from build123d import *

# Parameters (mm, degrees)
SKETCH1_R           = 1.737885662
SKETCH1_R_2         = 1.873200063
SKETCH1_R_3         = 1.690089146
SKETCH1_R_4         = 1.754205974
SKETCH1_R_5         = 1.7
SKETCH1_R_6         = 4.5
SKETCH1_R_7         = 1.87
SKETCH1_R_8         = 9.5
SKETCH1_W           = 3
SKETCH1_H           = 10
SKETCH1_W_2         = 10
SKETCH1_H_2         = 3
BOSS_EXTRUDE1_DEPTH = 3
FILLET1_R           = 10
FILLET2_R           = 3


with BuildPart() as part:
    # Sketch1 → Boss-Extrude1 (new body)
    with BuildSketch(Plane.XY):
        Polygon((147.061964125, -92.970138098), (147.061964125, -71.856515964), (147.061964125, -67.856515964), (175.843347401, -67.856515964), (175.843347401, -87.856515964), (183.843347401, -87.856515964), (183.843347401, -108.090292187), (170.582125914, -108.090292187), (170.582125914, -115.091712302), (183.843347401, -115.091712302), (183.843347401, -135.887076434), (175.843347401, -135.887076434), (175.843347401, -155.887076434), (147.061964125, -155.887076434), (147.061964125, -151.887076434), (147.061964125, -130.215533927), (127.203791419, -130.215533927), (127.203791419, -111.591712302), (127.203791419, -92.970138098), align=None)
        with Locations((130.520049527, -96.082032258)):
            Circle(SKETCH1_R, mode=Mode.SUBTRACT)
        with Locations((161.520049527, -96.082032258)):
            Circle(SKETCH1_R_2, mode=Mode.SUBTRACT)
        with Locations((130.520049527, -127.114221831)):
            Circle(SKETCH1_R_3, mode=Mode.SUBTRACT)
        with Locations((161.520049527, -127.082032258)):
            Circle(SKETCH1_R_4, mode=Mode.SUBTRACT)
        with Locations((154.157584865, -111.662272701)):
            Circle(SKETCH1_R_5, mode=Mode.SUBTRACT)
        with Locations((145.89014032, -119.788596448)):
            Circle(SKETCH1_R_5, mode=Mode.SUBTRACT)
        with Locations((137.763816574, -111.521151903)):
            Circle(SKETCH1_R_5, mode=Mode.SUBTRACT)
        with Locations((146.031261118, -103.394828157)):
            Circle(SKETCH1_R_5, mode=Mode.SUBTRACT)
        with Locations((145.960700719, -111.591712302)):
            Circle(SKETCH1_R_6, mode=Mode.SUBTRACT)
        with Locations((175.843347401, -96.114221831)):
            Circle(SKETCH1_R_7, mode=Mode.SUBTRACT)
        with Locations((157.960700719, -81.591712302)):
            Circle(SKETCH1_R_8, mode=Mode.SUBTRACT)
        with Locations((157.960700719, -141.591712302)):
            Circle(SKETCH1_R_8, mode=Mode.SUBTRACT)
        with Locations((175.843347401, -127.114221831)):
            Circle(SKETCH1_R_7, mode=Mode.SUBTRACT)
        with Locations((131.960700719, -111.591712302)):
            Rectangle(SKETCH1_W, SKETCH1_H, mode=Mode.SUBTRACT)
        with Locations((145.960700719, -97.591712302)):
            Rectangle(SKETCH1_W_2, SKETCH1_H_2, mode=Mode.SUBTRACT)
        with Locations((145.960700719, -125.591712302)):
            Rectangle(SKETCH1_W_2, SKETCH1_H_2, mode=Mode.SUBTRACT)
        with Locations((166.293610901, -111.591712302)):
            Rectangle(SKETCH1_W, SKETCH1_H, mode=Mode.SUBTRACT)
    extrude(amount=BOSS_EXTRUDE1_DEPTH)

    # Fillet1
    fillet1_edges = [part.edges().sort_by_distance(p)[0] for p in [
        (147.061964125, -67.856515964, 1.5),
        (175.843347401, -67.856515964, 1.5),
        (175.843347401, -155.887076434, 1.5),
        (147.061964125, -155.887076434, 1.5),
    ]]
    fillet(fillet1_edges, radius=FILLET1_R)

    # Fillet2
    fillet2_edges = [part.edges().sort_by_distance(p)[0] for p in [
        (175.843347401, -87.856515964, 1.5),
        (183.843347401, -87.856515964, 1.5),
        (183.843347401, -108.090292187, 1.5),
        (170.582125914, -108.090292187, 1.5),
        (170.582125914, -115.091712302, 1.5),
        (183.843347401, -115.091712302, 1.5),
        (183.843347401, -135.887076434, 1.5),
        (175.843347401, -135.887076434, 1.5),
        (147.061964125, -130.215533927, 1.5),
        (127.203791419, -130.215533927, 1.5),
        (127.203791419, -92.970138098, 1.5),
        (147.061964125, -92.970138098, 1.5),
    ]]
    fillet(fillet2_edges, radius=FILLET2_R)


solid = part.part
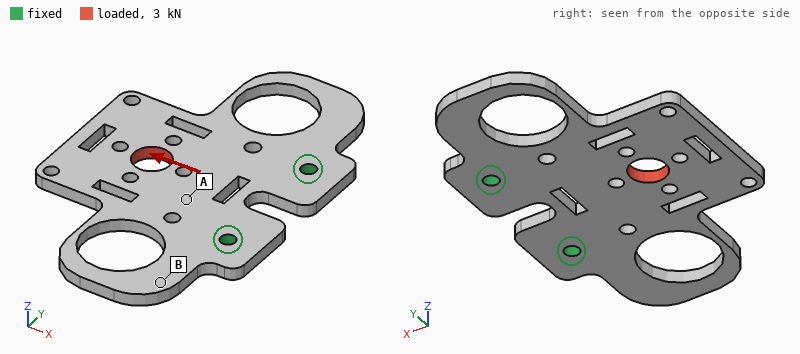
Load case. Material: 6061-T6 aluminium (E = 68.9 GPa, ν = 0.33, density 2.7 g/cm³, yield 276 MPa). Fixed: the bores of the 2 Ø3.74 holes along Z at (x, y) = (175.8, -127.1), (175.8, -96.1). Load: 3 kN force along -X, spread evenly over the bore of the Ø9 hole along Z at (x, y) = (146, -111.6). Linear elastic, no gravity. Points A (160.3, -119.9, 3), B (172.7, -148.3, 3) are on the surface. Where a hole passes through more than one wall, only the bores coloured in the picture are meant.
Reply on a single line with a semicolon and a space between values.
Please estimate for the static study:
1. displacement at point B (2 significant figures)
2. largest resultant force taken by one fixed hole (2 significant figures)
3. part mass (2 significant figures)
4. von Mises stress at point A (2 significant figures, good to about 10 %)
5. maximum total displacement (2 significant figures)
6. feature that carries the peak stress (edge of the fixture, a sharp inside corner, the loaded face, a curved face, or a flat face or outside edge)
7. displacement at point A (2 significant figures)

5.2 µm; 1.6 kN; 21 g; 40 MPa; 26 µm; a curved face; 10 µm
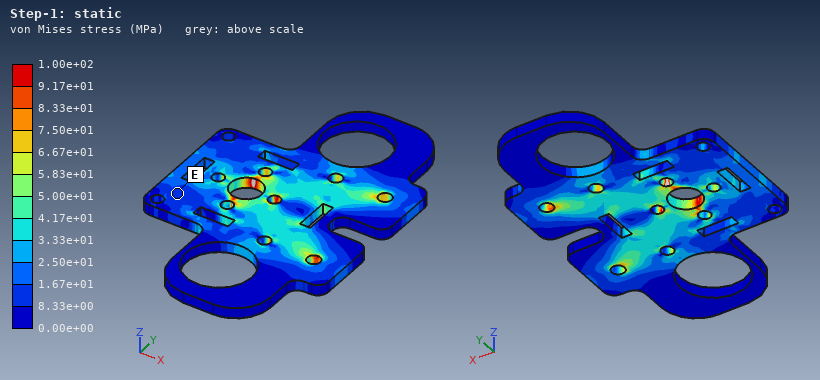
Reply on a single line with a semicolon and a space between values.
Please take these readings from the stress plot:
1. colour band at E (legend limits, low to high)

8.33e+00 to 1.67e+01 MPa
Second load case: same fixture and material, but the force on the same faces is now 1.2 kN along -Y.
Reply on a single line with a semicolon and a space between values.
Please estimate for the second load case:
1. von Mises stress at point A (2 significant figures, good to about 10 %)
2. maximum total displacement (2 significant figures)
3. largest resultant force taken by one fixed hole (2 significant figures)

18 MPa; 45 µm; 1.2 kN
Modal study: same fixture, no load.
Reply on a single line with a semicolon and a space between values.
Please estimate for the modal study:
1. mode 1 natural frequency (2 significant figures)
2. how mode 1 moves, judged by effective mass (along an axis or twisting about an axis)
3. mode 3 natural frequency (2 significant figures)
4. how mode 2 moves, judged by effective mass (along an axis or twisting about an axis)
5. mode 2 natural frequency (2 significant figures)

1100 Hz; along Z; 2700 Hz; twisting about X; 2300 Hz
